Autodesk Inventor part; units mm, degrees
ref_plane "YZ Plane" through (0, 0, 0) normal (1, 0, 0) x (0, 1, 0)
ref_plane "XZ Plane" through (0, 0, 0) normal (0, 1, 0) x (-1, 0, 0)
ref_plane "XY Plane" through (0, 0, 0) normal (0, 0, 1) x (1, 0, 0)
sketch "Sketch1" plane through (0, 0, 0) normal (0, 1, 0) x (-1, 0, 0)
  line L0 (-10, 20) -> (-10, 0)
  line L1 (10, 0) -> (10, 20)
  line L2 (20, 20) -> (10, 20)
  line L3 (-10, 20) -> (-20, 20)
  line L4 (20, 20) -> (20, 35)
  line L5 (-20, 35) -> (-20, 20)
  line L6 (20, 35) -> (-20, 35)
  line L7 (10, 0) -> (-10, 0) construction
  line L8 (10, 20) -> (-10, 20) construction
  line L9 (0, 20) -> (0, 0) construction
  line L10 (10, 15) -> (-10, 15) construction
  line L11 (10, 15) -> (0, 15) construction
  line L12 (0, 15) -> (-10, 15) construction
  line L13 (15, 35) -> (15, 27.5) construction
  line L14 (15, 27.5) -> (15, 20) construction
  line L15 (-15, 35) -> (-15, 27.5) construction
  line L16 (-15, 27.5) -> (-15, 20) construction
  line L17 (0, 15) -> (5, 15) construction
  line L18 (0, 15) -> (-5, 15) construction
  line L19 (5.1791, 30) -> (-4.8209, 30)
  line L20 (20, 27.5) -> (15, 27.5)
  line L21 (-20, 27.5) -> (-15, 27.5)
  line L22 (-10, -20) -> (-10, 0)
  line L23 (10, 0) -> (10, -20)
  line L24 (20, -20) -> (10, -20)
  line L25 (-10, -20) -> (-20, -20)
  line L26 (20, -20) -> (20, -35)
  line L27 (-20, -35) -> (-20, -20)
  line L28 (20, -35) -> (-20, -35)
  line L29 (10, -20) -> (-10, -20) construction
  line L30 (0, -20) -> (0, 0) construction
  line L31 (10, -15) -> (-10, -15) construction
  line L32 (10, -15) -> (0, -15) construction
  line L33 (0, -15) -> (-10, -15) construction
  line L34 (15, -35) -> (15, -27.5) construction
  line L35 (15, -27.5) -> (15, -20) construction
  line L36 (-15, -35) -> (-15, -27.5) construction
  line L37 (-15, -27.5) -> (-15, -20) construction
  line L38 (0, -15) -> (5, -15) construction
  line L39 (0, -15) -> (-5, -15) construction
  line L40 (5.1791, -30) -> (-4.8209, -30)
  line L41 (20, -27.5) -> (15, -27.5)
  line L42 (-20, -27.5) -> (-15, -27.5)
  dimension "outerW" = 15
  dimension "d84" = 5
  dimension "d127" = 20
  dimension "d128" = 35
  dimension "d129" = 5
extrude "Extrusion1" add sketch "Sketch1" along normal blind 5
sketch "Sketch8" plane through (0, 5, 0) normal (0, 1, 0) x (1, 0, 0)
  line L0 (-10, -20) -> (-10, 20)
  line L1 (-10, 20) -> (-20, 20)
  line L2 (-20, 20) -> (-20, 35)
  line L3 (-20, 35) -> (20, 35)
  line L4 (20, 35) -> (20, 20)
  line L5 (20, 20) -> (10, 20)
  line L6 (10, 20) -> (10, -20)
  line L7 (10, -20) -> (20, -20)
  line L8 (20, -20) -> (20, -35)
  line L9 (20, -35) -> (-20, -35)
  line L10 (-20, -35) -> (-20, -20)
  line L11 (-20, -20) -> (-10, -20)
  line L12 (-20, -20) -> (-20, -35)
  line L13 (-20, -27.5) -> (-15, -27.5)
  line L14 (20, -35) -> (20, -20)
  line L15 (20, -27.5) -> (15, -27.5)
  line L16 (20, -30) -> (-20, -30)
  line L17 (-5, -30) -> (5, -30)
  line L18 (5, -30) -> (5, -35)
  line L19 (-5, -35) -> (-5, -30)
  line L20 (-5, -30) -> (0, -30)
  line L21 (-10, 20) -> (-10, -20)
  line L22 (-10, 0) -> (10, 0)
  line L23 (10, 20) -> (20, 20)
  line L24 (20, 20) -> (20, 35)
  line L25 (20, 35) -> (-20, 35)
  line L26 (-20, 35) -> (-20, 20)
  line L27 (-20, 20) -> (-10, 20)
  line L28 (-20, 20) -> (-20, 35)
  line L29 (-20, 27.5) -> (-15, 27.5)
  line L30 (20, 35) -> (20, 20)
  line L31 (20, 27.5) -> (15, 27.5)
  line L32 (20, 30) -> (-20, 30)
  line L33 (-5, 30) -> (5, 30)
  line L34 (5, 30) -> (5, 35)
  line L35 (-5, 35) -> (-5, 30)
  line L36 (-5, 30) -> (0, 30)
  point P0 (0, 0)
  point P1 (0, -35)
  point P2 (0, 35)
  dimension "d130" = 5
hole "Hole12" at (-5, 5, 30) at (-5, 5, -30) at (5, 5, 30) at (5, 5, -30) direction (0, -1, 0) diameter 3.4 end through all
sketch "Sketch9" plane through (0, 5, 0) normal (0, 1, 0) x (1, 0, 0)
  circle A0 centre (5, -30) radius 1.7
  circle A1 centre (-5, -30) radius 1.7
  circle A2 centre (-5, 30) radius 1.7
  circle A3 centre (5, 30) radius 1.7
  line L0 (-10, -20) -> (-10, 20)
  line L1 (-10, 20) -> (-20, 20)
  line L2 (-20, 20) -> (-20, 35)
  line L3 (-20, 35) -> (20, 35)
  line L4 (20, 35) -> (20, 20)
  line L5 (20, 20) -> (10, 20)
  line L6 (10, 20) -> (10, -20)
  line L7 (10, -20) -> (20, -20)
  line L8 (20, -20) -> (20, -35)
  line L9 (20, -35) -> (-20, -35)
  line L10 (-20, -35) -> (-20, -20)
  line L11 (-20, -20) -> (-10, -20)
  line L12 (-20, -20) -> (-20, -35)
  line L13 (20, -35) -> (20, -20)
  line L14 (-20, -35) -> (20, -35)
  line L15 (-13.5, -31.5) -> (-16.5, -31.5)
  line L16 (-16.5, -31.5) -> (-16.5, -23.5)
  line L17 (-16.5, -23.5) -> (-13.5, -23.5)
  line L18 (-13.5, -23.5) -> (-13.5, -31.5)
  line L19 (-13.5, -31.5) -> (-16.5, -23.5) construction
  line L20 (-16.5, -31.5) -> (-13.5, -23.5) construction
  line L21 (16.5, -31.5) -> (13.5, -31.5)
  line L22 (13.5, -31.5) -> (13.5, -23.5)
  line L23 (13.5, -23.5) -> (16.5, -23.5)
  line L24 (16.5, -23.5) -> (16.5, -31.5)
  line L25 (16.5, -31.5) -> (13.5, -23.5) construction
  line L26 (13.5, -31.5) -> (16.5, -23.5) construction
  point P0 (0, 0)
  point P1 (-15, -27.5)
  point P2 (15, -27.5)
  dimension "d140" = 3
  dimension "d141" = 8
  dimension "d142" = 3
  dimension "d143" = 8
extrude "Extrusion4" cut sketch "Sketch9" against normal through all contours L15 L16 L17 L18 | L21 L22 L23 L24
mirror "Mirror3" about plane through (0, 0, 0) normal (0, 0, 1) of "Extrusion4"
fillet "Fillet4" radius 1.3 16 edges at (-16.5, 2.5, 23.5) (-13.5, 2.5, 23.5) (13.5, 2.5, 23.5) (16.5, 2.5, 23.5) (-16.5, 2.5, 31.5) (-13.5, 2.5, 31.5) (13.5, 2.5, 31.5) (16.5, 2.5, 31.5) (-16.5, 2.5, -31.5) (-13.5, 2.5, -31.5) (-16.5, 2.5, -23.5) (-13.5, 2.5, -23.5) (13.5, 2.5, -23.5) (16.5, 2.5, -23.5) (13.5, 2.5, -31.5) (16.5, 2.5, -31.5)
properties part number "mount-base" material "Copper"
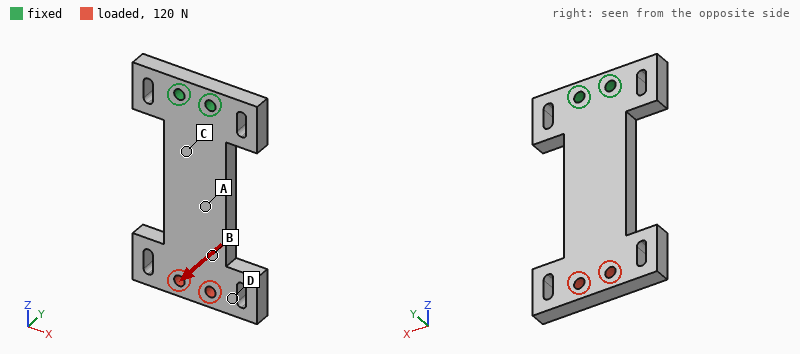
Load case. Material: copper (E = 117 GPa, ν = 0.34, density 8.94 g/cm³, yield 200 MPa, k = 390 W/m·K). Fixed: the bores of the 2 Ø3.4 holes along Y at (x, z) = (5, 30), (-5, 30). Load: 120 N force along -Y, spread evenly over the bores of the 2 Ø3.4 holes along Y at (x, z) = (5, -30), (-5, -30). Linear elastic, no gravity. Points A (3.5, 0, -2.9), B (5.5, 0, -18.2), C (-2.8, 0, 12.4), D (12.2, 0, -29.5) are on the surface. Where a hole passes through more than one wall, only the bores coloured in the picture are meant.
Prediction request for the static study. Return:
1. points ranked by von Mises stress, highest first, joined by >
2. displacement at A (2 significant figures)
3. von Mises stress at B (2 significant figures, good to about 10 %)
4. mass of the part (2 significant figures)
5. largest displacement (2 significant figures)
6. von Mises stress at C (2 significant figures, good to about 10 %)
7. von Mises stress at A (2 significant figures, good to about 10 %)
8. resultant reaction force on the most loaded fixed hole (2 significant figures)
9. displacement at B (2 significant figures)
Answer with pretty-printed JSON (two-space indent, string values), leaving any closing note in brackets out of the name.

{
  "points ranked by von Mises stress, highest first, joined by >": "C > A > B > D",
  "displacement at A": "0.12 mm",
  "von Mises stress at B": "17 MPa",
  "mass of the part": "84 g",
  "largest displacement": "0.36 mm",
  "von Mises stress at C": "59 MPa",
  "von Mises stress at A": "39 MPa",
  "resultant reaction force on the most loaded fixed hole": "60 N",
  "displacement at B": "0.23 mm"
}
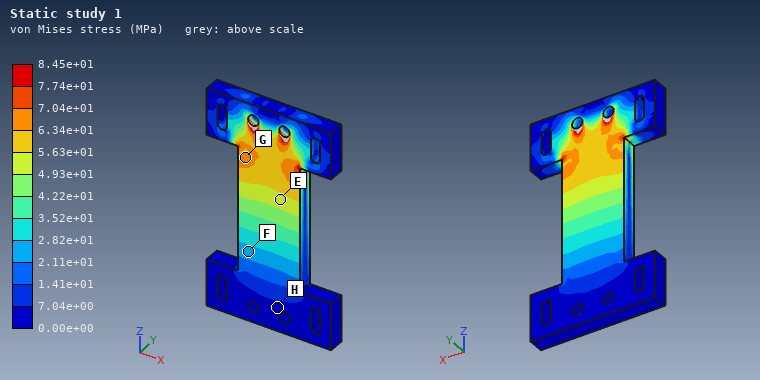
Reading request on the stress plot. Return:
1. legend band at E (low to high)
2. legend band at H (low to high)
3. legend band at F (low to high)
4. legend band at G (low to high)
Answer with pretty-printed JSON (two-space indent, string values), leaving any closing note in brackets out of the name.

{
  "legend band at E": "4.93e+01 to 5.63e+01 MPa",
  "legend band at H": "0.00e+00 to 7.04e+00 MPa",
  "legend band at F": "2.11e+01 to 2.82e+01 MPa",
  "legend band at G": "6.34e+01 to 7.04e+01 MPa"
}
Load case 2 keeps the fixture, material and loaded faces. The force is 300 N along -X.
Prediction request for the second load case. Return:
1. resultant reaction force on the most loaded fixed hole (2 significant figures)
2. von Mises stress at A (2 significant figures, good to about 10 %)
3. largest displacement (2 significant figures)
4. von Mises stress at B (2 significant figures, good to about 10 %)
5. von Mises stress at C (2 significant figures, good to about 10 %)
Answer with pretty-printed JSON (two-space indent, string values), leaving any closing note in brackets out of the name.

{
  "resultant reaction force on the most loaded fixed hole": "1.4 kN",
  "von Mises stress at A": "11 MPa",
  "largest displacement": "72 µm",
  "von Mises stress at B": "7.9 MPa",
  "von Mises stress at C": "12 MPa"
}
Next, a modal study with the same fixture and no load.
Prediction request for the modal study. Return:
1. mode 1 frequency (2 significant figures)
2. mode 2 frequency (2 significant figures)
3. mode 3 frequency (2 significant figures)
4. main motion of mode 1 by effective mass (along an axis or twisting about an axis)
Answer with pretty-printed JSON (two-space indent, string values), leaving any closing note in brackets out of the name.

{
  "mode 1 frequency": "590 Hz",
  "mode 2 frequency": "2100 Hz",
  "mode 3 frequency": "2100 Hz",
  "main motion of mode 1 by effective mass": "along Y"
}
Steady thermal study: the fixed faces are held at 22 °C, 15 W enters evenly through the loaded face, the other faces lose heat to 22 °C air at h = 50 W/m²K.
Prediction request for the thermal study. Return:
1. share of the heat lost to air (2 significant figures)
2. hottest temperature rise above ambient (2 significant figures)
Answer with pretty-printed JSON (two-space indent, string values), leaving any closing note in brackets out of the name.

{
  "share of the heat lost to air": "17 %",
  "hottest temperature rise above ambient": "19 K"
}
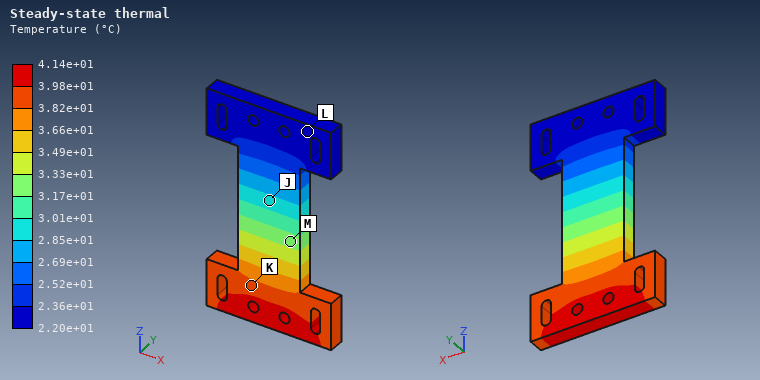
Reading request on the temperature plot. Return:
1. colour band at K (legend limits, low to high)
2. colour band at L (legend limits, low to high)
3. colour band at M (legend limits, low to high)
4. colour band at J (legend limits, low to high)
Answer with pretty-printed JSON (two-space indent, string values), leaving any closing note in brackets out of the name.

{
  "colour band at K": "3.82e+01 to 3.98e+01 °C",
  "colour band at L": "2.20e+01 to 2.36e+01 °C",
  "colour band at M": "3.17e+01 to 3.33e+01 °C",
  "colour band at J": "2.85e+01 to 3.01e+01 °C"
}
